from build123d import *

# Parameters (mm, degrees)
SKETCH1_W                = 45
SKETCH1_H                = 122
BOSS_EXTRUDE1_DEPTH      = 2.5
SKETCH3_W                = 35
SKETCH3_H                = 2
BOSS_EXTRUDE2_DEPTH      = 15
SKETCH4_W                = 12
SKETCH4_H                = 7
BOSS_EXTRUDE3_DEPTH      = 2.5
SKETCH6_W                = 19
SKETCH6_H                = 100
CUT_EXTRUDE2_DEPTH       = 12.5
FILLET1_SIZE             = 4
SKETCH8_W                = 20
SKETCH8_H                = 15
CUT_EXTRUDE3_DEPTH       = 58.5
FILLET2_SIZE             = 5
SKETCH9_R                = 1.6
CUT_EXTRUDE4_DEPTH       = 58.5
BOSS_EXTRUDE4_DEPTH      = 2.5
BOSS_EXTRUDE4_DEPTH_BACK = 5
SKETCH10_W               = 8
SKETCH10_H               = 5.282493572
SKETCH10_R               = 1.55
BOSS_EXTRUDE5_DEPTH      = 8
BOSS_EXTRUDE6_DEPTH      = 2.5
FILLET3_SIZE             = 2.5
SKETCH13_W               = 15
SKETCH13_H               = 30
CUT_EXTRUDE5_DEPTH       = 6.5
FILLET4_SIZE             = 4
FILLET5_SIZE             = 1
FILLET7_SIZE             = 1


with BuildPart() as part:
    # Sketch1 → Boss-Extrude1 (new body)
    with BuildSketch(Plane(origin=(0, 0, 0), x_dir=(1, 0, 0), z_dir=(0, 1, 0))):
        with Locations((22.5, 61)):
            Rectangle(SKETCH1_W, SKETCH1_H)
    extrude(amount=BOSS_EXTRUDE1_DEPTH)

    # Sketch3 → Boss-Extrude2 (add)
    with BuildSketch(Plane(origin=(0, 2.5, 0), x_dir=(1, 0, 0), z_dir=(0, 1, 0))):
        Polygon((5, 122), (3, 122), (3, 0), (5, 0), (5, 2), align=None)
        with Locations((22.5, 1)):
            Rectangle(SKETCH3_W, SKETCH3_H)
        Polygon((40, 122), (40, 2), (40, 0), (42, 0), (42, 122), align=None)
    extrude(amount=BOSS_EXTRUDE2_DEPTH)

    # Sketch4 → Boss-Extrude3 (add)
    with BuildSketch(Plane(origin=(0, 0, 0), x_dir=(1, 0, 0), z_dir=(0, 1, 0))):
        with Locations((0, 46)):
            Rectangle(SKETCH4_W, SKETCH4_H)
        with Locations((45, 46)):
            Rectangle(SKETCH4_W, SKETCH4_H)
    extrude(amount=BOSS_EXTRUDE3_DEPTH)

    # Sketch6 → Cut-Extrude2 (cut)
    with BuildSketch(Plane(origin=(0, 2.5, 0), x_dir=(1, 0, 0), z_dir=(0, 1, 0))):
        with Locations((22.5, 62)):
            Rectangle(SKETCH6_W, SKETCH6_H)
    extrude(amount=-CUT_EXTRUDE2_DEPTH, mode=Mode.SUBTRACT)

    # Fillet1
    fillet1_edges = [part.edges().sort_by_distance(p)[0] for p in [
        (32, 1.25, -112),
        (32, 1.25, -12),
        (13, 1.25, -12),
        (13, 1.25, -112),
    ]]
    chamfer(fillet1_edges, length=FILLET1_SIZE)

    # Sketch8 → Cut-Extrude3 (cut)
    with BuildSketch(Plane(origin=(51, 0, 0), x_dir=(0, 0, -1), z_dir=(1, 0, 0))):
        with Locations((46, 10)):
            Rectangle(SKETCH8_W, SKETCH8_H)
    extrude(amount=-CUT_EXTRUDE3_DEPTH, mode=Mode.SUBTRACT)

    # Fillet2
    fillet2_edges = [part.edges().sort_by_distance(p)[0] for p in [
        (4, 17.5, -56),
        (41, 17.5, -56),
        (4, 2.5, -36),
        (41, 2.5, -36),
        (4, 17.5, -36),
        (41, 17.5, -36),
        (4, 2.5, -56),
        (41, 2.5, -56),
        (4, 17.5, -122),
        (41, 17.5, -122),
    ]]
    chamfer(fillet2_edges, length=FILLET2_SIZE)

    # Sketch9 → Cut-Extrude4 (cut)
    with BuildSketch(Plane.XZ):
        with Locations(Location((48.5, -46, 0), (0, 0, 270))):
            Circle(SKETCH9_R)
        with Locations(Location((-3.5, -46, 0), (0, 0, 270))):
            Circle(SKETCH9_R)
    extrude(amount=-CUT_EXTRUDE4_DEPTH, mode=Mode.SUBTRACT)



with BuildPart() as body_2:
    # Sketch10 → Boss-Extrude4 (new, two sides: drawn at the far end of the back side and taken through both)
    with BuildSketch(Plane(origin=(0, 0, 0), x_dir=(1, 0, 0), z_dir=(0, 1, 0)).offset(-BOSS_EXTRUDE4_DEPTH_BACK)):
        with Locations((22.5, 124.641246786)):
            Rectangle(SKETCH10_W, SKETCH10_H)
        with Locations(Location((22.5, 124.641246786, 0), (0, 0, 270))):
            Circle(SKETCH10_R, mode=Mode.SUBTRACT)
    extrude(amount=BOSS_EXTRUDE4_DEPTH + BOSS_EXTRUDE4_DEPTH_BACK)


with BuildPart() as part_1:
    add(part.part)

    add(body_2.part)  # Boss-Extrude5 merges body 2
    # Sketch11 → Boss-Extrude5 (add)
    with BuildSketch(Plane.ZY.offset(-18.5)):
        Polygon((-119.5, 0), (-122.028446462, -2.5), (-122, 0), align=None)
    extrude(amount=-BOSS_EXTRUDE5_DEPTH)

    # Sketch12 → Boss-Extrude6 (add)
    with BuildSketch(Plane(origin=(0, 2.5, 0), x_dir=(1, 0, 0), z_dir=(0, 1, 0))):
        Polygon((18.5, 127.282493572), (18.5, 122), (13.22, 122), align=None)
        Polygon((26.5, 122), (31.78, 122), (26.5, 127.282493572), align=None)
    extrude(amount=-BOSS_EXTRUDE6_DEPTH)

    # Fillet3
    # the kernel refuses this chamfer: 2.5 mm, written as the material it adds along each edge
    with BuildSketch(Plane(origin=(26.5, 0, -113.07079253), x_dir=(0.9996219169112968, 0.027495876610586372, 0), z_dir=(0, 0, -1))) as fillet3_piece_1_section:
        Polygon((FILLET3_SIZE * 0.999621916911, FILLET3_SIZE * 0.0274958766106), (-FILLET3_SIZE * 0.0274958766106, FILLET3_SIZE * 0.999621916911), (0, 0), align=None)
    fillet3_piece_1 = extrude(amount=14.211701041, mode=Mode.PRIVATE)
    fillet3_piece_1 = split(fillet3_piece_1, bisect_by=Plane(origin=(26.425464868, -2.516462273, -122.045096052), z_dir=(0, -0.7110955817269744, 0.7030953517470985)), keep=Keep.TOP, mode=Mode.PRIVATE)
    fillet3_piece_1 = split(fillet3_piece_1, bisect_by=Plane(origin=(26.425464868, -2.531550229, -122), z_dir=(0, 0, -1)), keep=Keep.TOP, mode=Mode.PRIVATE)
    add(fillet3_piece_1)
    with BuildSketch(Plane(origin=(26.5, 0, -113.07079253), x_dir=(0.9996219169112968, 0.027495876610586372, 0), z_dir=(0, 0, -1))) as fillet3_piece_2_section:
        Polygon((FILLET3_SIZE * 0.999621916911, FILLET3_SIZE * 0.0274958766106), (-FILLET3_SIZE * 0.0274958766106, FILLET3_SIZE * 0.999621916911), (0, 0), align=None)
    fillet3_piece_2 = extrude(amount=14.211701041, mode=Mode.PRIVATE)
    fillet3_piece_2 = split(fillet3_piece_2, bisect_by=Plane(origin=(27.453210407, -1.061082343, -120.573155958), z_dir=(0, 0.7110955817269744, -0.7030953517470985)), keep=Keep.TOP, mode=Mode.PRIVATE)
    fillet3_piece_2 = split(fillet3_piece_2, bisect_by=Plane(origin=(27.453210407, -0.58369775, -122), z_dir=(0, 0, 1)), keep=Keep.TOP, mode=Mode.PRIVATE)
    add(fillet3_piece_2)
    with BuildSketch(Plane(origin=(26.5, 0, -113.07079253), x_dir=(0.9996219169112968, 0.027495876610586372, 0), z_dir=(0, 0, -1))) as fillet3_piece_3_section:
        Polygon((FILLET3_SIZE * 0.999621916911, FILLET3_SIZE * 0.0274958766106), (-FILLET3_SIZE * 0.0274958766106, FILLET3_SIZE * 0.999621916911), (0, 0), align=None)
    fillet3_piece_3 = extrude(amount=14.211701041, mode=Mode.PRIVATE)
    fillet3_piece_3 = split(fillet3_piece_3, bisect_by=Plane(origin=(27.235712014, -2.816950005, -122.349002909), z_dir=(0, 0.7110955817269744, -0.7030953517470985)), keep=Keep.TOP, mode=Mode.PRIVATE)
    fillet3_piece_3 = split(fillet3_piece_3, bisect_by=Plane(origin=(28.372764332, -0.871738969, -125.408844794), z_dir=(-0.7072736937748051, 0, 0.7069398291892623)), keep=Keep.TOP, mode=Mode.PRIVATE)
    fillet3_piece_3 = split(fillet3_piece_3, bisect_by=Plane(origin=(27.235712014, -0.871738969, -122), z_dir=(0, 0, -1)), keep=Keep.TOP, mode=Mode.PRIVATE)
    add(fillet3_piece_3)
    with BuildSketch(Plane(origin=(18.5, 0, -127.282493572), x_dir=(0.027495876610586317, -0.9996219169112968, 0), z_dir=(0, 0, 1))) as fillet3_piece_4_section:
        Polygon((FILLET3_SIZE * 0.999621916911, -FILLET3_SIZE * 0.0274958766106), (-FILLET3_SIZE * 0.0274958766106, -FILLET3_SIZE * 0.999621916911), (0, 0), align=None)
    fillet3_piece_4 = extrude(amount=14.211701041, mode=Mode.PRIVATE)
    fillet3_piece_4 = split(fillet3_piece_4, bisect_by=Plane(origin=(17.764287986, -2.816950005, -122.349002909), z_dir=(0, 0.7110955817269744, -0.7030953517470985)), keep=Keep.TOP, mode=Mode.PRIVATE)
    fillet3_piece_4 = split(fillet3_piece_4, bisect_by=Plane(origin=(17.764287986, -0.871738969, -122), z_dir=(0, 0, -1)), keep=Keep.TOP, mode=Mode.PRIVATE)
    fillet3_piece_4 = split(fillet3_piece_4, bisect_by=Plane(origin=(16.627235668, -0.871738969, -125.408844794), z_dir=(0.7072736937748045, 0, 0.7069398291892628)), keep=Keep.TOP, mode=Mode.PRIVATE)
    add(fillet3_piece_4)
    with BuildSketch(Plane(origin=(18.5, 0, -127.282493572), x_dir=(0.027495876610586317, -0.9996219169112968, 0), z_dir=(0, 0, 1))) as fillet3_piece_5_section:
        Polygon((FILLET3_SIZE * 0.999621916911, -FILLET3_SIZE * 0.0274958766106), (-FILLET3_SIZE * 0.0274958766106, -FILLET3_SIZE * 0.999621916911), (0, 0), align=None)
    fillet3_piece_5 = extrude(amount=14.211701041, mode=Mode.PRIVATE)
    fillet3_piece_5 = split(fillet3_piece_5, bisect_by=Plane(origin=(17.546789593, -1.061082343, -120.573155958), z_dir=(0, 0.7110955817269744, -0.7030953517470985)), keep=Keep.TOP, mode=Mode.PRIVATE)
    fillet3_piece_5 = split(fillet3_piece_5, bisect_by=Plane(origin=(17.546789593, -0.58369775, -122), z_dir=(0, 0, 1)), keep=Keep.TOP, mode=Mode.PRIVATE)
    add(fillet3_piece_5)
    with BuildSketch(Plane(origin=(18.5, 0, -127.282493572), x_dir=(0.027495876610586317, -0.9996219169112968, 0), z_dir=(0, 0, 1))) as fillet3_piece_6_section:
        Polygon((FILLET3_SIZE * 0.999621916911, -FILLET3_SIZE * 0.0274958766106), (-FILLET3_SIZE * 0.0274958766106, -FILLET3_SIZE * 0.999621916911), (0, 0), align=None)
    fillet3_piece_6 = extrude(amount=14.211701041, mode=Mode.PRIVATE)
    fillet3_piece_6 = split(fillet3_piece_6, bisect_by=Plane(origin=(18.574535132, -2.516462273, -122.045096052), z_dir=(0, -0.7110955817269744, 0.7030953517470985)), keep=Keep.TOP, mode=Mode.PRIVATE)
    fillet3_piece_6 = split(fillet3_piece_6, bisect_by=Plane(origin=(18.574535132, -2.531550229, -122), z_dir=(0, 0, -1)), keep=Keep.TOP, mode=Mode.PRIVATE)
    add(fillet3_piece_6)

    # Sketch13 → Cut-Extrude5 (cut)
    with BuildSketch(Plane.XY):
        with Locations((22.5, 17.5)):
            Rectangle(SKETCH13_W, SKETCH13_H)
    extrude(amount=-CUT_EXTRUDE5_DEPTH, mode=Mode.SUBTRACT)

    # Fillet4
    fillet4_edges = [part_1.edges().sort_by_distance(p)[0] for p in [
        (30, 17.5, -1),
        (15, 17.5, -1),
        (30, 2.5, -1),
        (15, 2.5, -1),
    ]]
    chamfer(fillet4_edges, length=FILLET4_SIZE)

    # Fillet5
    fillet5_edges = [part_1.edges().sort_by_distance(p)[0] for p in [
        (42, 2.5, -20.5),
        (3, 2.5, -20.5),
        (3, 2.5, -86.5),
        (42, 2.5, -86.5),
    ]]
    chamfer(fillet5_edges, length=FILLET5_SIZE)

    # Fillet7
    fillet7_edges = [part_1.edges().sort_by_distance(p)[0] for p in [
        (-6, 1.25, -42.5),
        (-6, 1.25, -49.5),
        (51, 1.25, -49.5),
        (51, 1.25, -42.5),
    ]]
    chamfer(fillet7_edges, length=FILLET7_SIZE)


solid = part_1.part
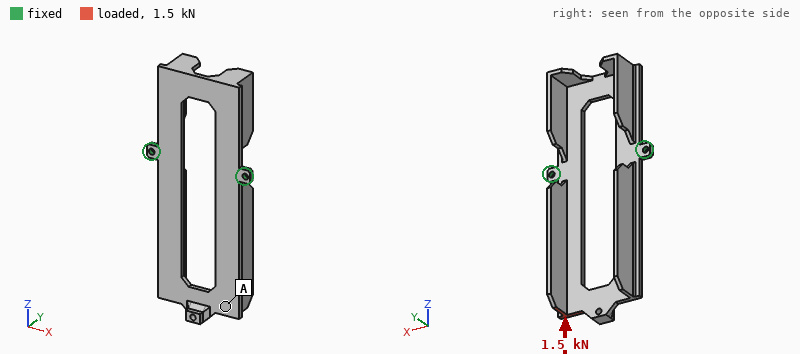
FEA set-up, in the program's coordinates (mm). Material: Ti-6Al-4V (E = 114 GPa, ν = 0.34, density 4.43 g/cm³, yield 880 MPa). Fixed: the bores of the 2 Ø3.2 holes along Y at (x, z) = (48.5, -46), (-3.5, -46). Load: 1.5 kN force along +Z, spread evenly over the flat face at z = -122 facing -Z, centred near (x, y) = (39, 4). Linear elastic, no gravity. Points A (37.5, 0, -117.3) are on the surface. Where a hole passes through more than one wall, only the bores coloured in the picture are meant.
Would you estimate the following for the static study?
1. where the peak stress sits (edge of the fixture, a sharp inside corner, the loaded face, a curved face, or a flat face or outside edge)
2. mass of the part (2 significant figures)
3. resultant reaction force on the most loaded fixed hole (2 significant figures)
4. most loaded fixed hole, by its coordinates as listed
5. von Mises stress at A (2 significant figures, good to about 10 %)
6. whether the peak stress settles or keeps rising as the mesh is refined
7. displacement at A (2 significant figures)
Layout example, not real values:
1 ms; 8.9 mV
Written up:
edge of the fixture; 73 g; 1.3 kN; (48.5, -46); 34 MPa; keeps rising; 0.94 mm
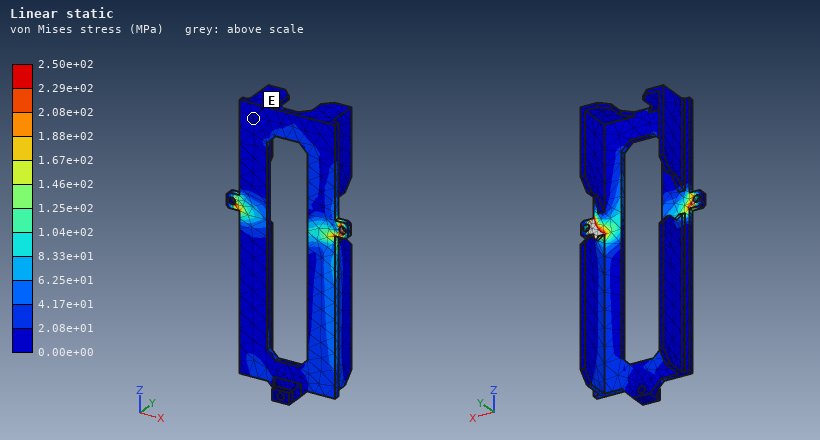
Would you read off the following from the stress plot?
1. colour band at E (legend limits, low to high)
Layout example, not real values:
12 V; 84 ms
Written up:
0.00e+00 to 2.08e+01 MPa
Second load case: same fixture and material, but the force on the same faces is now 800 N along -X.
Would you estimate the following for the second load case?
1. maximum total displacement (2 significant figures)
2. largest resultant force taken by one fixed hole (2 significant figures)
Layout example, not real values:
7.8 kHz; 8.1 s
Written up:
0.70 mm; 1.3 kN
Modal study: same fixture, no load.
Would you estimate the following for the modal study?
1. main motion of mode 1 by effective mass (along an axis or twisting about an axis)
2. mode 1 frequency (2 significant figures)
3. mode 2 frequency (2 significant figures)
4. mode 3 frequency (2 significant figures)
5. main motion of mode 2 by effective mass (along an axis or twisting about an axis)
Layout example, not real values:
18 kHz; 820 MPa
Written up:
along Y; 260 Hz; 610 Hz; 800 Hz; along Y
